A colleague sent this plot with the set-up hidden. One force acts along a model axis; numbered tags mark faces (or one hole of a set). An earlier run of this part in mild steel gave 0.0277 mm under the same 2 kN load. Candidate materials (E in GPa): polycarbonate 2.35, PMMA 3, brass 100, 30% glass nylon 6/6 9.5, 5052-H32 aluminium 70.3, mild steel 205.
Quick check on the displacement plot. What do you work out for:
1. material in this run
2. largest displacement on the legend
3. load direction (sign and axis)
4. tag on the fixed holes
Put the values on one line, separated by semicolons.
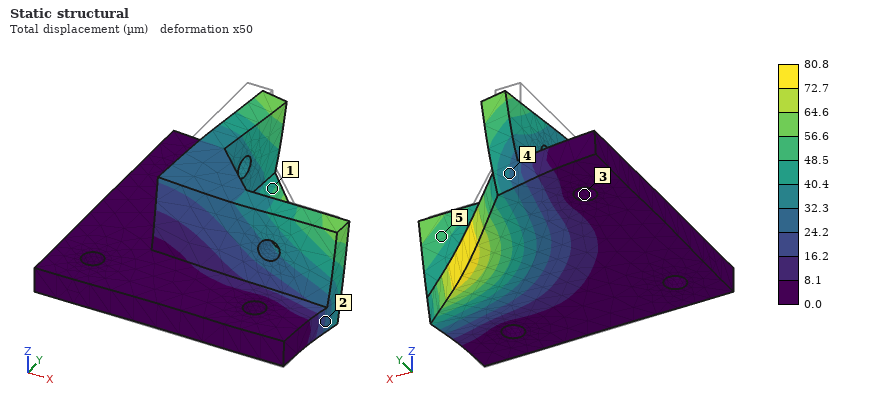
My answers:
5052-H32 aluminium; 80.8 µm; -Z; 3
